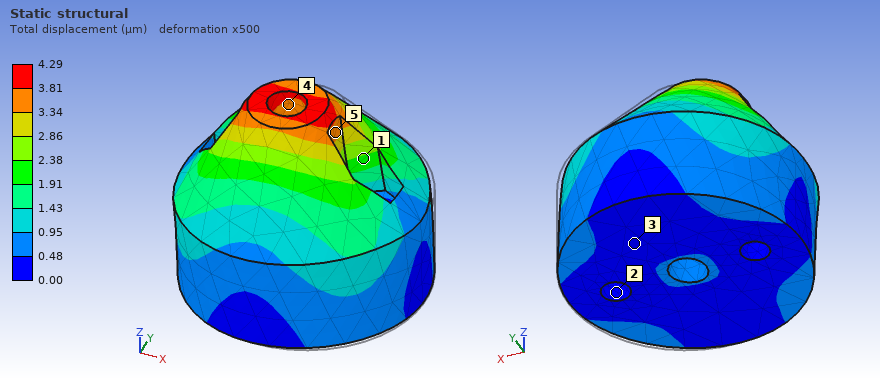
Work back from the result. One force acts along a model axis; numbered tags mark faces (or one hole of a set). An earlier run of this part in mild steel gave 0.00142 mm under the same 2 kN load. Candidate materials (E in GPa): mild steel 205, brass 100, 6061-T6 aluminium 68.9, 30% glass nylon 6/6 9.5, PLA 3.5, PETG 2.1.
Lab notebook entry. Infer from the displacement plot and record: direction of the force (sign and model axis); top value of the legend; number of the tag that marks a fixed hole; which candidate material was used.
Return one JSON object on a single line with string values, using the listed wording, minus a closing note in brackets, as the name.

{"direction of the force": "-X", "top value of the legend": "4.29 µm", "number of the tag that marks a fixed hole": "2", "which candidate material was used": "6061-T6 aluminium"}
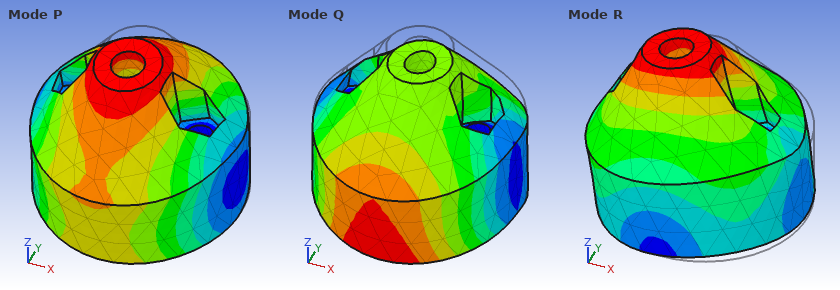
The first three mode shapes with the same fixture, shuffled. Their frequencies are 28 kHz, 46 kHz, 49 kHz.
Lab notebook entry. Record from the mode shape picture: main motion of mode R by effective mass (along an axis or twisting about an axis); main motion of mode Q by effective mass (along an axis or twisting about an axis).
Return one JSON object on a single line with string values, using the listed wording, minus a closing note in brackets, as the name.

{"main motion of mode R by effective mass": "along X", "main motion of mode Q by effective mass": "along Z"}
